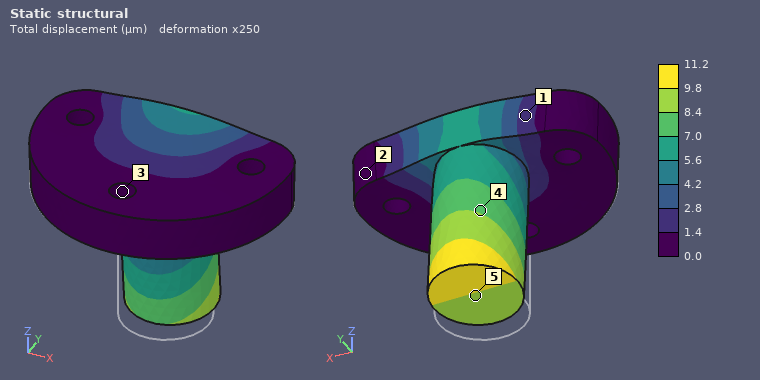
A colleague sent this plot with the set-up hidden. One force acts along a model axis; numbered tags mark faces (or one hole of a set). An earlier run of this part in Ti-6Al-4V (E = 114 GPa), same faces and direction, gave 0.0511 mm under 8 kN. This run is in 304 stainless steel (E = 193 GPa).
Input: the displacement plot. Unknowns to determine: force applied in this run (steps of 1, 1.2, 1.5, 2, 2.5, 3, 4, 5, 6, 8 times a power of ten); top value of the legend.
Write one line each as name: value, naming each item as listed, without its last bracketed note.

force applied in this run: 3 kN
top value of the legend: 11.2 µm
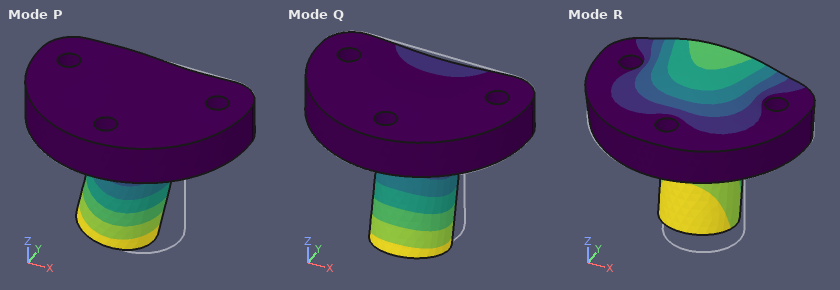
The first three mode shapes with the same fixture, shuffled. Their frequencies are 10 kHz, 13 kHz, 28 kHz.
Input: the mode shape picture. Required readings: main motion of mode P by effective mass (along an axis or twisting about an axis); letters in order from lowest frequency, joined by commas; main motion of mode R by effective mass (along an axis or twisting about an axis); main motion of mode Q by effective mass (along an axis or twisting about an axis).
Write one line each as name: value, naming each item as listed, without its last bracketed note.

main motion of mode P by effective mass: along X
letters in order from lowest frequency, joined by commas: Q, P, R
main motion of mode R by effective mass: along Z
main motion of mode Q by effective mass: along Y
